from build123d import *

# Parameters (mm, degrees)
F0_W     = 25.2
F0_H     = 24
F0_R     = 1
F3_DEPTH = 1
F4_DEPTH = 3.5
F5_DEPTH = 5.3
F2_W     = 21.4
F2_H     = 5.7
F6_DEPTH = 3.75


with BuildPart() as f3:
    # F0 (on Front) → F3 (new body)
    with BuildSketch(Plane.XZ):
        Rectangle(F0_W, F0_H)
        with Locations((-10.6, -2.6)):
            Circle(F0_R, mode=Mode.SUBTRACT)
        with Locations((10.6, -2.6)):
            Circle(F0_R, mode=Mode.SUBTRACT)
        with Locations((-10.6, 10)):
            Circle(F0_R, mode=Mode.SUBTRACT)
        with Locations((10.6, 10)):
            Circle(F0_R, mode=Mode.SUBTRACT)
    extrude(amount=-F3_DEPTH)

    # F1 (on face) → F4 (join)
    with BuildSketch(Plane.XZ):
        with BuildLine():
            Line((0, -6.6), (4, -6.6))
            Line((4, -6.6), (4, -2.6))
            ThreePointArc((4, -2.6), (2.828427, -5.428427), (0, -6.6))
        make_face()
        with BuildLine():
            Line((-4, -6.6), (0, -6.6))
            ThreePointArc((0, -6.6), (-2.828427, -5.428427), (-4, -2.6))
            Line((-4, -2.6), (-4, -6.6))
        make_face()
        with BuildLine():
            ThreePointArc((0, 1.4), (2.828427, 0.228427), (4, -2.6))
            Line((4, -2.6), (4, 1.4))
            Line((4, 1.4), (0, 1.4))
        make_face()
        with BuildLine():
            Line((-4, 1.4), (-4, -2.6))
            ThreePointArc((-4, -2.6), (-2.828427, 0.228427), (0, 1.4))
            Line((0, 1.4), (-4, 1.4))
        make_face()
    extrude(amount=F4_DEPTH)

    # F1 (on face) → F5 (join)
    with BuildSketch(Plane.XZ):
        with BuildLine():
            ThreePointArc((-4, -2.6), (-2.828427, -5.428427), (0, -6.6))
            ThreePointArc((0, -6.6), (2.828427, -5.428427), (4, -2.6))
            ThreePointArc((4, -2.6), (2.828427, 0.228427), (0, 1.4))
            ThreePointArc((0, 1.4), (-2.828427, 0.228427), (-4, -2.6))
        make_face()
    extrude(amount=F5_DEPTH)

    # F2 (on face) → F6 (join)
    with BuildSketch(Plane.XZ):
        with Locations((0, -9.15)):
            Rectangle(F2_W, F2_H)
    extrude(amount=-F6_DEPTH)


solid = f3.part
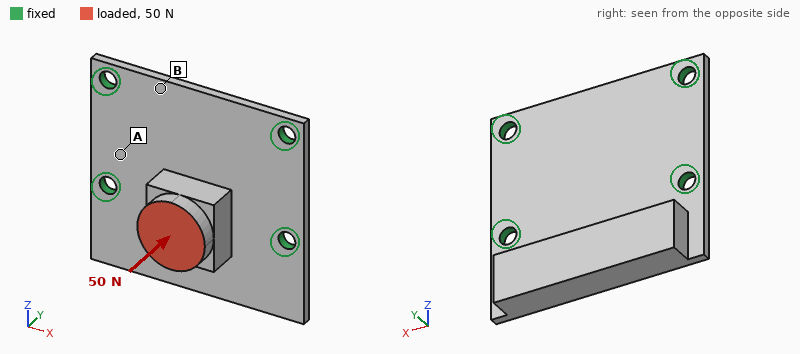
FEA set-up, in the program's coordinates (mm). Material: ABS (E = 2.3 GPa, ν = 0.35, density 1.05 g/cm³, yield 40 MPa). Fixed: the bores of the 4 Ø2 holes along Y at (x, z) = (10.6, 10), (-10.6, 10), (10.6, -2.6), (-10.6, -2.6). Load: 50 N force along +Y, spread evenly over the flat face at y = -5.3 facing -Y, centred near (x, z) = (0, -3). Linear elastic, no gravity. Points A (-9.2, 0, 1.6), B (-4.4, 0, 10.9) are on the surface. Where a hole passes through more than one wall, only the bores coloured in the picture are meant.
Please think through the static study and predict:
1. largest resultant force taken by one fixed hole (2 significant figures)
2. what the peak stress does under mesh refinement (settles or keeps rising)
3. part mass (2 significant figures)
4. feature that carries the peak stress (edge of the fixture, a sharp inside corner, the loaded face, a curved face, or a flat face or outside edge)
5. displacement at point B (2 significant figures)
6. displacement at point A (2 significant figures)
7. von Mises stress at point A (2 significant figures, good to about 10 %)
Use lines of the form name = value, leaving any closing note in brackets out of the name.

largest resultant force taken by one fixed hole = 23 N
what the peak stress does under mesh refinement = keeps rising
part mass = 1.3 g
feature that carries the peak stress = edge of the fixture
displacement at point B = 0.050 mm
displacement at point A = 0.042 mm
von Mises stress at point A = 5.8 MPa
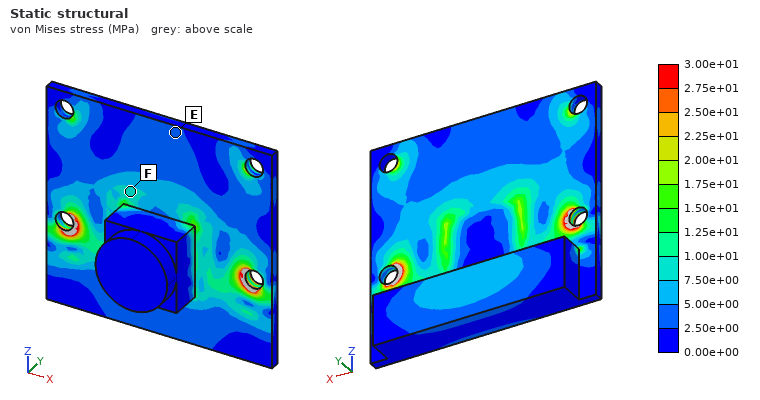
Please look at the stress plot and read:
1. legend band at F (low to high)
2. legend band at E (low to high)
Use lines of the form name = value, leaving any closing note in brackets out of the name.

legend band at F = 7.50e+00 to 1.00e+01 MPa
legend band at E = 2.50e+00 to 5.00e+00 MPa
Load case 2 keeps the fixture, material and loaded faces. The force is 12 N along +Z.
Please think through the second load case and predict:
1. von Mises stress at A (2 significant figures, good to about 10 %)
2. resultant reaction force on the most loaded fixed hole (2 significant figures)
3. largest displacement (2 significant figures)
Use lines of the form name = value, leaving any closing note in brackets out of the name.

von Mises stress at A = 2.5 MPa
resultant reaction force on the most loaded fixed hole = 5.0 N
largest displacement = 0.15 mm
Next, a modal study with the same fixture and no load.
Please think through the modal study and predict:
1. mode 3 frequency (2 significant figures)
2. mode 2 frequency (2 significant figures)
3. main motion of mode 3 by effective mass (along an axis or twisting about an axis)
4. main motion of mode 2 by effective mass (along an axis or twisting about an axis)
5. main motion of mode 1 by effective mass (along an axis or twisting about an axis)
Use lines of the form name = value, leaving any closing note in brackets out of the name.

mode 3 frequency = 5100 Hz
mode 2 frequency = 3200 Hz
main motion of mode 3 by effective mass = twisting about Z
main motion of mode 2 by effective mass = along Y
main motion of mode 1 by effective mass = along Y
